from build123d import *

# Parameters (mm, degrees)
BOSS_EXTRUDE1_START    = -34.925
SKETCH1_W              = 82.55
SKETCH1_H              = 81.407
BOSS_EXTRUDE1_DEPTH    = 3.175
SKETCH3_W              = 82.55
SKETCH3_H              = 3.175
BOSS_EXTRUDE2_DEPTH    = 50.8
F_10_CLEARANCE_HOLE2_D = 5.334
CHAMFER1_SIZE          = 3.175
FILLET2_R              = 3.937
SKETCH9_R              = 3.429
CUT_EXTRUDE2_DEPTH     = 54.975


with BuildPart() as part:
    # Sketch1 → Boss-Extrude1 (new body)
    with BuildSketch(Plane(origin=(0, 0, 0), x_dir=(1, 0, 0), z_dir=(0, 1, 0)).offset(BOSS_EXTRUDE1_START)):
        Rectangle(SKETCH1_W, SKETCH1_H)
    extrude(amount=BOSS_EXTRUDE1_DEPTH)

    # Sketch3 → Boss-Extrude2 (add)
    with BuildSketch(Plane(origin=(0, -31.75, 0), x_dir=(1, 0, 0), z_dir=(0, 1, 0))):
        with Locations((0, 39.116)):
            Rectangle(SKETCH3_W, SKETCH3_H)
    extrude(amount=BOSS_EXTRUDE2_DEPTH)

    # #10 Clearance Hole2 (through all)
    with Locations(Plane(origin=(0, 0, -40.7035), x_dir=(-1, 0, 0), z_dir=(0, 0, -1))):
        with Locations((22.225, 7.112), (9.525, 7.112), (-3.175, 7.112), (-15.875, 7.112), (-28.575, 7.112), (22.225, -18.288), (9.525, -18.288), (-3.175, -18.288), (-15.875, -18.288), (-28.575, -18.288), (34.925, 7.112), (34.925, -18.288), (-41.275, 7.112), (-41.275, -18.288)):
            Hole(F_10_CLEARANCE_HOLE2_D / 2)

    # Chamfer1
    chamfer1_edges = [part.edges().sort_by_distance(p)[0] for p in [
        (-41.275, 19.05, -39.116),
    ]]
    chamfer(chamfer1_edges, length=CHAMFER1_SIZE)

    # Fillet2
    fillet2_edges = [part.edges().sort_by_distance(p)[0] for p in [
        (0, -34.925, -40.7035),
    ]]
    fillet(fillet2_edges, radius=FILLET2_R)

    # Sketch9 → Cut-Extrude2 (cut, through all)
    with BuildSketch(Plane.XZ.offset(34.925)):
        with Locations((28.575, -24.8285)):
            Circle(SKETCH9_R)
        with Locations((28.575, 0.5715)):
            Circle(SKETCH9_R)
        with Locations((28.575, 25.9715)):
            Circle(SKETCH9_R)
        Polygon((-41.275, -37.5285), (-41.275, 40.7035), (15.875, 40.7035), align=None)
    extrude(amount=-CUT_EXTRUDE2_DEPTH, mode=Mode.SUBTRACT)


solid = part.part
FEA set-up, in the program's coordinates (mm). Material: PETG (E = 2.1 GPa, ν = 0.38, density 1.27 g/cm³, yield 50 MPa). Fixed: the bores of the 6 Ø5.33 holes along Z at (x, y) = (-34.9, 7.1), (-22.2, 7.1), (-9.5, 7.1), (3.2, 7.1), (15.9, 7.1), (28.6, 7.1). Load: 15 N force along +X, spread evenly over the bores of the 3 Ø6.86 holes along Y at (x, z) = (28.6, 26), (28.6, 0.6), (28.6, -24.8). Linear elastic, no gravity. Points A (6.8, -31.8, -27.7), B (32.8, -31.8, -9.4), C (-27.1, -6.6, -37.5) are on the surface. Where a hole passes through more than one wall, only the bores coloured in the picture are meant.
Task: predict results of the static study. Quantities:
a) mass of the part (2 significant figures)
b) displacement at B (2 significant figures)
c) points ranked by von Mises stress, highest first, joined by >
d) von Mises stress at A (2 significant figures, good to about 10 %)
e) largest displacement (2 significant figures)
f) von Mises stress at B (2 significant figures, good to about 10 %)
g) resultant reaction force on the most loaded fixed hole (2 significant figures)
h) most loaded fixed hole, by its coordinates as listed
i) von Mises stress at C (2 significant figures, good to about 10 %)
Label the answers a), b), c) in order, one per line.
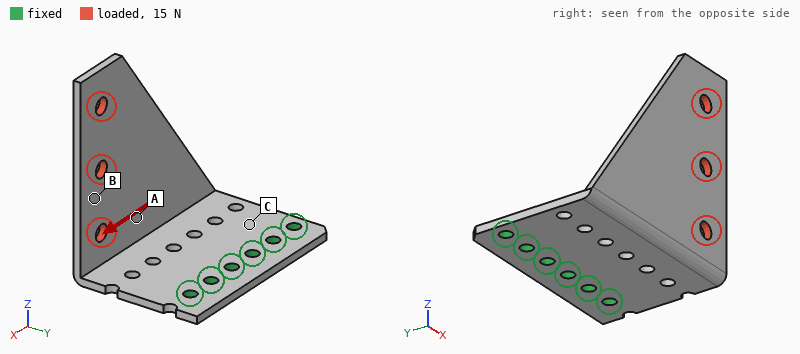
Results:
a) 33 g
b) 0.68 mm
c) C > A > B
d) 1.1 MPa
e) 1.4 mm
f) 0.54 MPa
g) 12 N
h) (28.6, 7.1)
i) 2.1 MPa
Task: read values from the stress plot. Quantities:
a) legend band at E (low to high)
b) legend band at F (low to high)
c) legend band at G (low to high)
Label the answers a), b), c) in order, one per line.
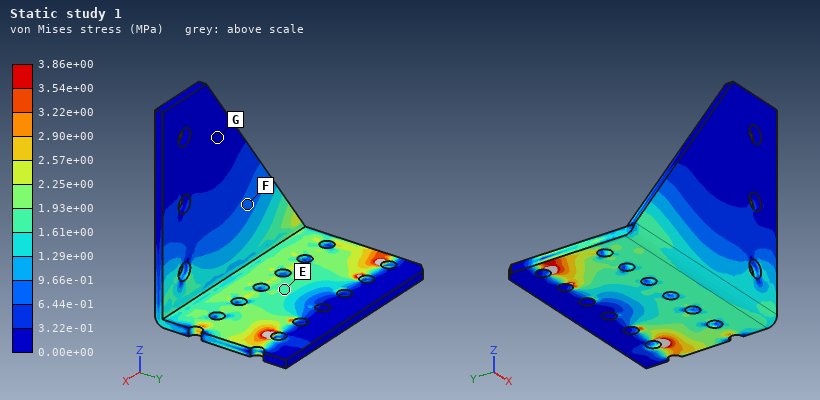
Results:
a) 1.61e+00 to 1.93e+00 MPa
b) 6.44e-01 to 9.66e-01 MPa
c) 0.00e+00 to 3.22e-01 MPa
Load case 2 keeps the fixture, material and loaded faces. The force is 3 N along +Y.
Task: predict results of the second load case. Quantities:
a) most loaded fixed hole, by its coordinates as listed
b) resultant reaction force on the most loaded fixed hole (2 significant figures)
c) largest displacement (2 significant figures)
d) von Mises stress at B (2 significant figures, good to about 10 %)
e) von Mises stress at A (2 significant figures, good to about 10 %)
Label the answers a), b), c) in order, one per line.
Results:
a) (28.6, 7.1)
b) 1.8 N
c) 1.5 mm
d) 0.48 MPa
e) 0.78 MPa
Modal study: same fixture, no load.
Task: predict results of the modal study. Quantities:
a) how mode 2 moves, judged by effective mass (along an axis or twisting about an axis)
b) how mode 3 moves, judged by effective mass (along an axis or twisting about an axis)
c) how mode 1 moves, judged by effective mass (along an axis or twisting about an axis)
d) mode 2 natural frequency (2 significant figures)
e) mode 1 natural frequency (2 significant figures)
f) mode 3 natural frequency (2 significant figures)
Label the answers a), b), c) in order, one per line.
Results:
a) along X
b) along Z
c) along Y
d) 170 Hz
e) 79 Hz
f) 250 Hz
